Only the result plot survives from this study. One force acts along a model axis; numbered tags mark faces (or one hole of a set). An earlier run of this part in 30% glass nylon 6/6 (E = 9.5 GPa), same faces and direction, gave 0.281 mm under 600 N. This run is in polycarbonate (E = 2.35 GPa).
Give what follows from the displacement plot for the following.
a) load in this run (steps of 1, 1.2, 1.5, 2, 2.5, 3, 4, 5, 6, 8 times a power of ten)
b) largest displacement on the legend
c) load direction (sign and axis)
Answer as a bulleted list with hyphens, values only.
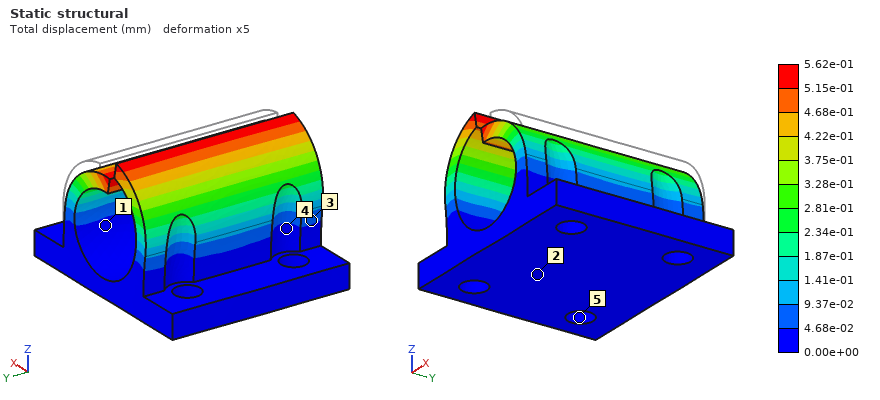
- 300 N
- 5.62e-01 mm
- -X
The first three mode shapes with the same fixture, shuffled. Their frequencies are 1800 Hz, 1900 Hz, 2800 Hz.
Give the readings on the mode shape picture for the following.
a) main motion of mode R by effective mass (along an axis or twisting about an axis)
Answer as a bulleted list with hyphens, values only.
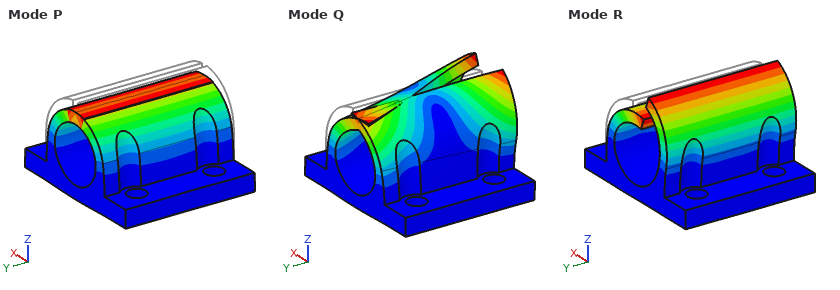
- along X
